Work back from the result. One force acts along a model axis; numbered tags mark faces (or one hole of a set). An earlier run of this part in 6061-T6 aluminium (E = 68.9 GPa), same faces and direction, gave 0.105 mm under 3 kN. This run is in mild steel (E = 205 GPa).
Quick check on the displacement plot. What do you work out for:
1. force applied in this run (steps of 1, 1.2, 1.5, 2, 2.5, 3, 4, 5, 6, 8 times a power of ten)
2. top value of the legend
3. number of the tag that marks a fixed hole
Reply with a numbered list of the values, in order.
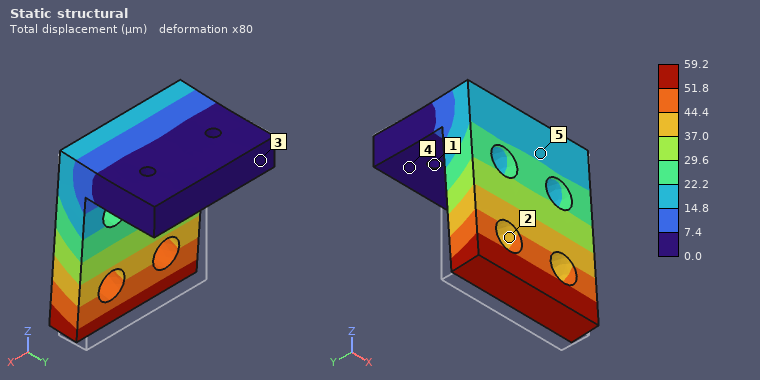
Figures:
1. 5 kN
2. 59.2 µm
3. 1
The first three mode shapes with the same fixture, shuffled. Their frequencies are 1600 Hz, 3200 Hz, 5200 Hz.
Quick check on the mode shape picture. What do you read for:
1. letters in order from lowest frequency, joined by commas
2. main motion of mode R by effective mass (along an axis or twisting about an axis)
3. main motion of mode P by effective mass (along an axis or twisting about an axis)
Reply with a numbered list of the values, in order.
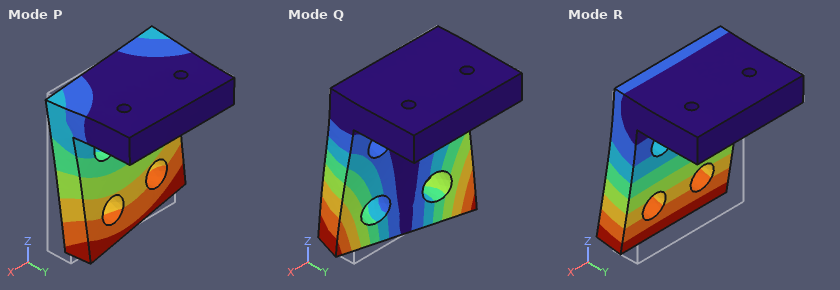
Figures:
1. R, P, Q
2. along Y
3. along X
